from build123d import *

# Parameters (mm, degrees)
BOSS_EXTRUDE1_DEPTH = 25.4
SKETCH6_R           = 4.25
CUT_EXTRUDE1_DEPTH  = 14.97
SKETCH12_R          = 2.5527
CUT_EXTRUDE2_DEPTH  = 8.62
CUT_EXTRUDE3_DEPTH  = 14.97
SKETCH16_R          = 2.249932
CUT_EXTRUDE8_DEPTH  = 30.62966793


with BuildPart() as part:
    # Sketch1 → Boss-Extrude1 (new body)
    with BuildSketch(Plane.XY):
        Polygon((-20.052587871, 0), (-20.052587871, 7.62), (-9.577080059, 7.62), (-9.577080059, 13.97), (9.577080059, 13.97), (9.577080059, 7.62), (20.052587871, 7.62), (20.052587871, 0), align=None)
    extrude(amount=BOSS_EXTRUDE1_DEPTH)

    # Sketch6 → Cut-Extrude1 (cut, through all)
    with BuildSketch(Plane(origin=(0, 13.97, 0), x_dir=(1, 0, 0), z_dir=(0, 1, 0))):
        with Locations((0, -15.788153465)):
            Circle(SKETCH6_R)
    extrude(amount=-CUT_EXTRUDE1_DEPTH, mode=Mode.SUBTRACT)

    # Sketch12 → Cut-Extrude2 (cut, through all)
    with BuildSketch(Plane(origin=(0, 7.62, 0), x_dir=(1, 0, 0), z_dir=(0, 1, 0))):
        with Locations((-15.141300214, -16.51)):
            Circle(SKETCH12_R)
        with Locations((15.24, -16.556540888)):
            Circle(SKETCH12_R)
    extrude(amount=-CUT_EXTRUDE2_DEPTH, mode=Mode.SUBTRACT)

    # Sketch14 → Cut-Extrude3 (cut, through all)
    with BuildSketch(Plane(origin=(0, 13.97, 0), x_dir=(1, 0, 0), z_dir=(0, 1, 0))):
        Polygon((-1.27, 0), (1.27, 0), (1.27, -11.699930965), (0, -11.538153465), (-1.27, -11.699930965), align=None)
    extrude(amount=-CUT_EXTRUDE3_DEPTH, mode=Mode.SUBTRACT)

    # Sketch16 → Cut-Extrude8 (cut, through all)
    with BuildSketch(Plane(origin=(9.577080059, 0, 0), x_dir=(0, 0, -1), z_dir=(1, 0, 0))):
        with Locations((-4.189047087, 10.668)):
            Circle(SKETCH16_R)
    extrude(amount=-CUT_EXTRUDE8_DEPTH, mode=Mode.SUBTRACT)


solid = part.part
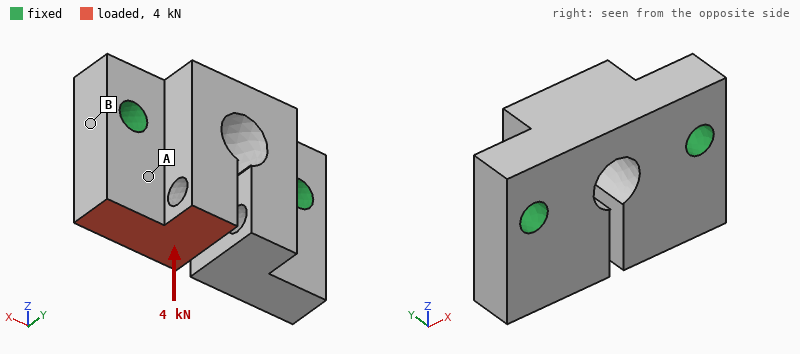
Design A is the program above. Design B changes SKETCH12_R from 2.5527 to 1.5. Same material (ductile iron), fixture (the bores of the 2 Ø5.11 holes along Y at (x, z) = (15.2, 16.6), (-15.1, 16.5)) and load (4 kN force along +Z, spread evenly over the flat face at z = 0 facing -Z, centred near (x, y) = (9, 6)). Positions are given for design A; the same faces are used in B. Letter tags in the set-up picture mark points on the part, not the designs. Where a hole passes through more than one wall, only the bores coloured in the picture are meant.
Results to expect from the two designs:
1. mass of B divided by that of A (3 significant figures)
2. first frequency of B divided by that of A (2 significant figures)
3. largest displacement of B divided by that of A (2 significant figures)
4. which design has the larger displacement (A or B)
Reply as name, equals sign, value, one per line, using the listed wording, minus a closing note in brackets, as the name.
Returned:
mass of B divided by that of A = 1.02
first frequency of B divided by that of A = 0.83
largest displacement of B divided by that of A = 1.3
which design has the larger displacement = B
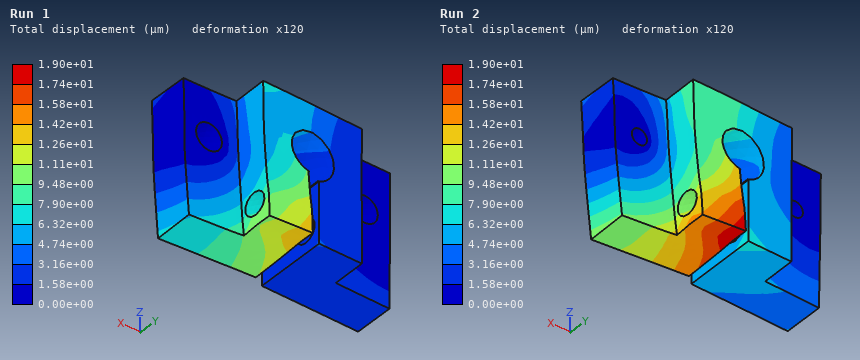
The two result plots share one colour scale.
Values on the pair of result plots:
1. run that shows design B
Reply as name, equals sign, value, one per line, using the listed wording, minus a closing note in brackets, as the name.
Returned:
run that shows design B = Run 2
